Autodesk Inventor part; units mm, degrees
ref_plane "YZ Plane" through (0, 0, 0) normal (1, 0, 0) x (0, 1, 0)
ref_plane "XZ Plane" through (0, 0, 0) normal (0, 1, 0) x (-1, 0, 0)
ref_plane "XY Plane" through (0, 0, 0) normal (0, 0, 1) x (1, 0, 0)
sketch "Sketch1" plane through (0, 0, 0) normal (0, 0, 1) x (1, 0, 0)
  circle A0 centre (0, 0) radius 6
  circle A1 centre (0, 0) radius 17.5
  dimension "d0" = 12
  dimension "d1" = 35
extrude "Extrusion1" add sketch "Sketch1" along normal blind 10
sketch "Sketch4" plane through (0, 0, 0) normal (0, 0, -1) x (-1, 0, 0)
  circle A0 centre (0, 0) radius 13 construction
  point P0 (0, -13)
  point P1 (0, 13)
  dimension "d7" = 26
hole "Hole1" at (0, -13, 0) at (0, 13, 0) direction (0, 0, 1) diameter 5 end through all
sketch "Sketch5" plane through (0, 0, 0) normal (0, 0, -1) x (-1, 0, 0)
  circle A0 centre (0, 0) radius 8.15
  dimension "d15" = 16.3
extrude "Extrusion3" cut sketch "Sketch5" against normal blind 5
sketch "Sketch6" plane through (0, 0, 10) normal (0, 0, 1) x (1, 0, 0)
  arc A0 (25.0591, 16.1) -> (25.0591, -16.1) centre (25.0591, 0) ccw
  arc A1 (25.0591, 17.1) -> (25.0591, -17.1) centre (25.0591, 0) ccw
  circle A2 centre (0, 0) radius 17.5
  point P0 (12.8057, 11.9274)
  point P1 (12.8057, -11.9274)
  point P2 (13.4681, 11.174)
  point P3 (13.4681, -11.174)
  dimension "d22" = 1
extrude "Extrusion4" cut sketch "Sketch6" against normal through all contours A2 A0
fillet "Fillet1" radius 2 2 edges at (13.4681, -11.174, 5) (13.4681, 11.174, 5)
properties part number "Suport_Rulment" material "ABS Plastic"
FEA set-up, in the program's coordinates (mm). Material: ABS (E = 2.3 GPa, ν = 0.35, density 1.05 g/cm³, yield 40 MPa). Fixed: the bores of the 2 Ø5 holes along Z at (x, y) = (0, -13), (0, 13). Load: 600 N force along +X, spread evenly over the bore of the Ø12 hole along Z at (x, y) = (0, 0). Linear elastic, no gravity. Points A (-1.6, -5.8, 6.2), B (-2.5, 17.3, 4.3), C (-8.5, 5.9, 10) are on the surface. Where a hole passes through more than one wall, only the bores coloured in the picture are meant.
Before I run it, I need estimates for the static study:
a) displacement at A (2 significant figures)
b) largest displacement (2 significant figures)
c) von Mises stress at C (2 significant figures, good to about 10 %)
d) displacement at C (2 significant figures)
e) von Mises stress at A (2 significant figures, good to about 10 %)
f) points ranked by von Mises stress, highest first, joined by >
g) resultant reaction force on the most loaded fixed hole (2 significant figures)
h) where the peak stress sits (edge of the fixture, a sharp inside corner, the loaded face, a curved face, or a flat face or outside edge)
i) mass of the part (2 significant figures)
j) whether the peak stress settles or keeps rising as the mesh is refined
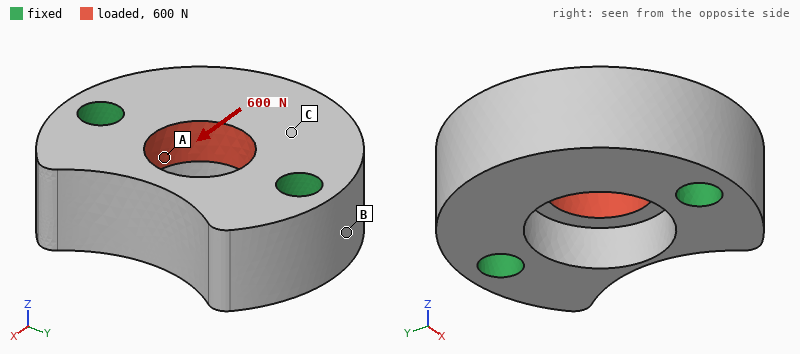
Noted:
21 µm
63 µm
3.2 MPa
23 µm
5.6 MPa
A > C > B
300 N
edge of the fixture
6.6 g
keeps rising
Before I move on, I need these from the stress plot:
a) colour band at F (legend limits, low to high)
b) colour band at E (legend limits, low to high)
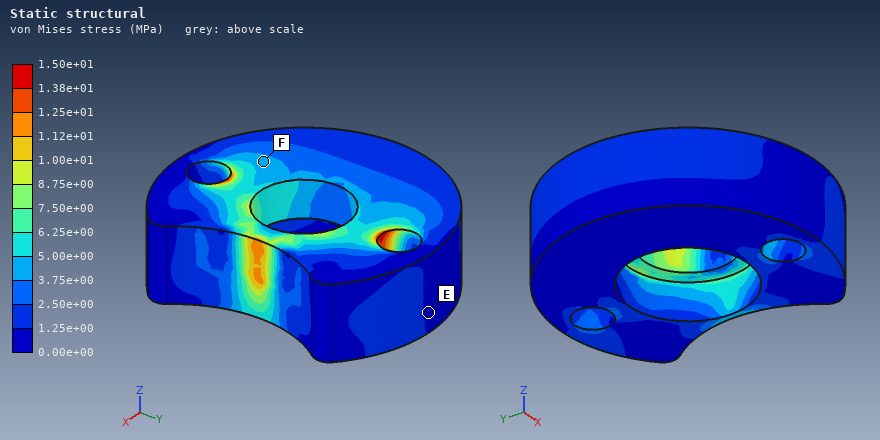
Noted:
3.75e+00 to 5.00e+00 MPa
0.00e+00 to 1.25e+00 MPa
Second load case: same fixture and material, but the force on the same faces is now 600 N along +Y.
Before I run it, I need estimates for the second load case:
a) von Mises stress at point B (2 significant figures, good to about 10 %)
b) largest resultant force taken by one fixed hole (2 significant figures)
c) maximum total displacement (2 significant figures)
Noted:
1.5 MPa
300 N
25 µm
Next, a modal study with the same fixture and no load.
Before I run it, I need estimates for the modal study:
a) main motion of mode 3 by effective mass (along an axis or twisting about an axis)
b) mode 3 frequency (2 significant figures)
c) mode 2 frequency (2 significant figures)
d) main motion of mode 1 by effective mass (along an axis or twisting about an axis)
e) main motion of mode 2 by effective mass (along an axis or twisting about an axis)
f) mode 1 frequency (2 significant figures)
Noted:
along Z
12 kHz
12 kHz
along Z
along Y
6600 Hz
